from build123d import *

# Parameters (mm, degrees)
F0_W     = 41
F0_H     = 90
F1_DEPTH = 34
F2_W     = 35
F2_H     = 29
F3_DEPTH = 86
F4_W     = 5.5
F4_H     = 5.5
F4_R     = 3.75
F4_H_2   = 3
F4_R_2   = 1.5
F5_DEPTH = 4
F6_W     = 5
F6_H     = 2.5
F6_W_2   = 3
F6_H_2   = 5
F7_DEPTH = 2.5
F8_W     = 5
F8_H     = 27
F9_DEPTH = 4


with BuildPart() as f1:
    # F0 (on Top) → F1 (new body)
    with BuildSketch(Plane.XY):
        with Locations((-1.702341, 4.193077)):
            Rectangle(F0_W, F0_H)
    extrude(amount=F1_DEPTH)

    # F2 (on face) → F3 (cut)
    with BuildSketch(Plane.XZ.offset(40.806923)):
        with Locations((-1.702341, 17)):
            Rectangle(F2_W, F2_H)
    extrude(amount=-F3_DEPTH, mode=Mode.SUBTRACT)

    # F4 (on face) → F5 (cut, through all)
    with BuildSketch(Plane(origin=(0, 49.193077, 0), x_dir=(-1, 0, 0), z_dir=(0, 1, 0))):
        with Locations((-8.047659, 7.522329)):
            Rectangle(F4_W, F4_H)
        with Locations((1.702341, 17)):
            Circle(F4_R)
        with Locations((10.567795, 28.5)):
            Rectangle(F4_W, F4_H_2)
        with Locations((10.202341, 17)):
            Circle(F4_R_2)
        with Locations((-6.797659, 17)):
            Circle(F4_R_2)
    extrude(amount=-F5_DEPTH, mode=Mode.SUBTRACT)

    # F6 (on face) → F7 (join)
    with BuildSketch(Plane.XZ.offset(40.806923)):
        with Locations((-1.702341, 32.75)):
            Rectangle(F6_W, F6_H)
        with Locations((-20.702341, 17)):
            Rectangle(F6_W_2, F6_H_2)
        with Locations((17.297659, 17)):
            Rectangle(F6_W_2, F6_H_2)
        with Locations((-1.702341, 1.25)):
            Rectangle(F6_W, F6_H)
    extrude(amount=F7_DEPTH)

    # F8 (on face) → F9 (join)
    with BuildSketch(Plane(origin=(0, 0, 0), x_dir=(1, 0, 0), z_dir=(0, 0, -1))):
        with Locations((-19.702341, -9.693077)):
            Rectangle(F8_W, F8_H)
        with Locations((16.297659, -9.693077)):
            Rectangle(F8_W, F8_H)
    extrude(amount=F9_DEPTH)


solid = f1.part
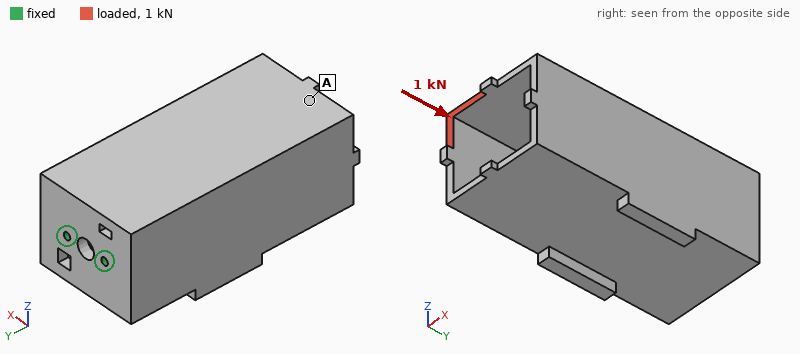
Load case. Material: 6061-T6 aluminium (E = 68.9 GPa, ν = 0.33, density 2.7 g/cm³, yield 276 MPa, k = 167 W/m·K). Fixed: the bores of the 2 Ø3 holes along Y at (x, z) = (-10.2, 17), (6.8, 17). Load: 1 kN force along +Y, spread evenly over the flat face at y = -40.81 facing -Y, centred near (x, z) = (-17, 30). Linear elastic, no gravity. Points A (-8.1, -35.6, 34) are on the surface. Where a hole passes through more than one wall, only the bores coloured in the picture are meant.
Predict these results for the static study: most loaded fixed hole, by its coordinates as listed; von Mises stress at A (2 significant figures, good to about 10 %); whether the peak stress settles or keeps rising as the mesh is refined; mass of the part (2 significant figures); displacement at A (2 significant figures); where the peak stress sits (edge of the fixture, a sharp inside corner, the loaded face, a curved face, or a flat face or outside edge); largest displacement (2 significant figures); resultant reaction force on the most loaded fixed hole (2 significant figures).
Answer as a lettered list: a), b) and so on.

a) (-10.2, 17)
b) 13 MPa
c) keeps rising
d) 110 g
e) 0.33 mm
f) edge of the fixture
g) 0.36 mm
h) 1.1 kN
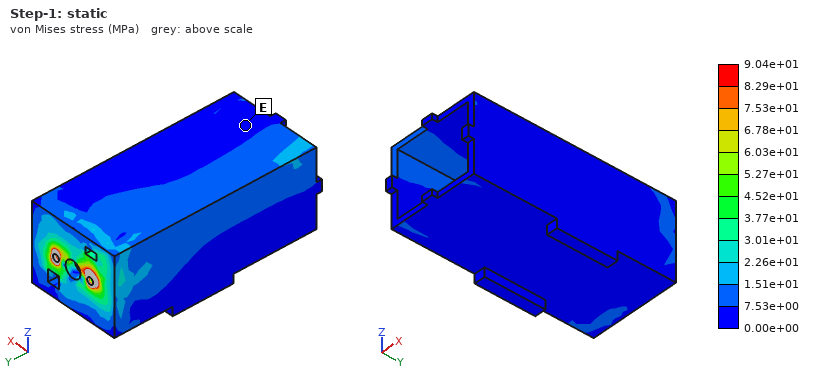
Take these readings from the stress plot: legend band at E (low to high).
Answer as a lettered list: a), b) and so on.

a) 0.00e+00 to 7.53e+00 MPa
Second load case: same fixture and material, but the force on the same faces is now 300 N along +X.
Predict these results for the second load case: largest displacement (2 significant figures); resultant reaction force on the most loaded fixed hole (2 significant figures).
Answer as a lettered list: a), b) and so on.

a) 0.22 mm
b) 1.1 kN
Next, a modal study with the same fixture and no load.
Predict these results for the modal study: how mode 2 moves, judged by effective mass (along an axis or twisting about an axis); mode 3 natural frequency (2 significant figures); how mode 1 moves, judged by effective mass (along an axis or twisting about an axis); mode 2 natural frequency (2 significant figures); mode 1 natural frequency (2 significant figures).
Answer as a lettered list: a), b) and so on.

a) along X
b) 3200 Hz
c) along Z
d) 1100 Hz
e) 590 Hz
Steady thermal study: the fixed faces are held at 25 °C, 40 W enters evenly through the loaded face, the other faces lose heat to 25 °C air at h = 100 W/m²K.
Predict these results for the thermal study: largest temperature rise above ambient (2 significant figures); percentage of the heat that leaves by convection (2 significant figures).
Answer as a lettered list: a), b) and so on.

a) 65 K
b) 80 %
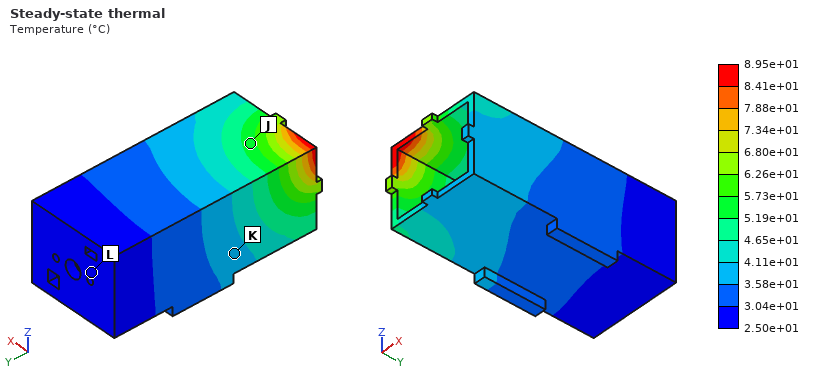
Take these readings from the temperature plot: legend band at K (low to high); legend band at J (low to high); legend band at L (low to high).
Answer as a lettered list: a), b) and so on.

a) 3.58e+01 to 4.11e+01 °C
b) 5.19e+01 to 5.73e+01 °C
c) 2.50e+01 to 3.04e+01 °C
